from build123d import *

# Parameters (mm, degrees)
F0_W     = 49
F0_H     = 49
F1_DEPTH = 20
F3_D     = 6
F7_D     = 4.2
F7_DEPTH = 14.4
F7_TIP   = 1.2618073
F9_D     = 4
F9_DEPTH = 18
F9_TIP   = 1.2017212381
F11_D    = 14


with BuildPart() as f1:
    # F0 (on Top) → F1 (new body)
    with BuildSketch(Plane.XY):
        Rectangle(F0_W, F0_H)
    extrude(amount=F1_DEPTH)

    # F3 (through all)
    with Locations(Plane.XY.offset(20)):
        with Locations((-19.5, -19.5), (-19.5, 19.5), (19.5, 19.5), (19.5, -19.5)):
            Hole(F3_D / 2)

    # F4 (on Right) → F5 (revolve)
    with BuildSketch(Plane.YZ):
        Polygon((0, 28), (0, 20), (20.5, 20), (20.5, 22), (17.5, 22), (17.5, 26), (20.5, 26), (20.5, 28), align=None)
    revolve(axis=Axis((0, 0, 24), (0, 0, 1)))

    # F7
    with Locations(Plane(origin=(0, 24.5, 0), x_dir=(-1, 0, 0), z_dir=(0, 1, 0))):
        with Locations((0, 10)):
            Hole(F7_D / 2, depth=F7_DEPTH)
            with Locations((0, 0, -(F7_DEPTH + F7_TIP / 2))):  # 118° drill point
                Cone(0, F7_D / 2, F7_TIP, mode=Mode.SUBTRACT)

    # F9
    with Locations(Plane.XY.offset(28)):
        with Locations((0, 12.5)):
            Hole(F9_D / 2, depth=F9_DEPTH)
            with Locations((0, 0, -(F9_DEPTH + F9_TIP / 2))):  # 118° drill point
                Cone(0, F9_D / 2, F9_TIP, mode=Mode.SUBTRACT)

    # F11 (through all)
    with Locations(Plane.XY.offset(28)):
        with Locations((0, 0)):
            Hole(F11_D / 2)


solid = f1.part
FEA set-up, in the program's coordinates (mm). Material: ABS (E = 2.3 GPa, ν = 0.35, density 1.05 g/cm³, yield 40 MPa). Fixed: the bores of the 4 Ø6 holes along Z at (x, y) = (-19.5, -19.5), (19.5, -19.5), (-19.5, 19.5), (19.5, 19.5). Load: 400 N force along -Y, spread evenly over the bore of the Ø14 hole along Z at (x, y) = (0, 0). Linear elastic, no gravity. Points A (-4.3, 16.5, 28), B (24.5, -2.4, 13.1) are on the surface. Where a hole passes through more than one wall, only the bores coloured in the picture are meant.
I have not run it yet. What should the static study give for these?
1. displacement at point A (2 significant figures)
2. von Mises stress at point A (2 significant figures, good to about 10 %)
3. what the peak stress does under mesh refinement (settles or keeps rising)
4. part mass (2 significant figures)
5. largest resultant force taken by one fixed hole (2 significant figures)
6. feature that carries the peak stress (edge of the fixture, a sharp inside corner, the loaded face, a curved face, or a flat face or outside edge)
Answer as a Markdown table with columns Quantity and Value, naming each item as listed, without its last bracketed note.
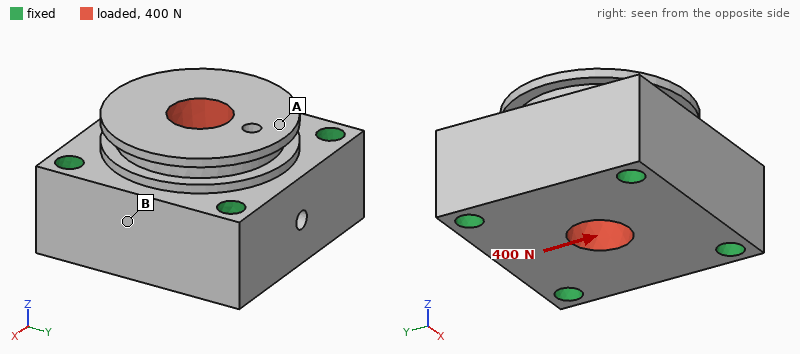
| Quantity | Value |
|---|---|
| displacement at point A | 5.3 µm |
| von Mises stress at point A | 0.29 MPa |
| what the peak stress does under mesh refinement | keeps rising |
| part mass | 53 g |
| largest resultant force taken by one fixed hole | 110 N |
| feature that carries the peak stress | edge of the fixture |
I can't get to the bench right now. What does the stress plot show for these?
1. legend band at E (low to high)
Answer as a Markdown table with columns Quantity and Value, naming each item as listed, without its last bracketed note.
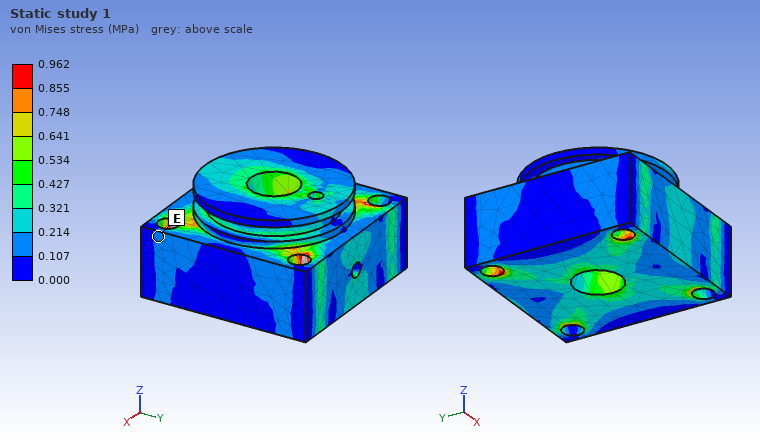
| Quantity | Value |
|---|---|
| legend band at E | 0.107 to 0.214 MPa |
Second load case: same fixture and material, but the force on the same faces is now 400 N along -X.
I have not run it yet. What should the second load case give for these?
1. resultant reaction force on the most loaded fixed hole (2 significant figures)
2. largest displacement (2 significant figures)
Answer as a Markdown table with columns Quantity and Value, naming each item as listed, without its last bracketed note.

| Quantity | Value |
|---|---|
| resultant reaction force on the most loaded fixed hole | 120 N |
| largest displacement | 6.6 µm |
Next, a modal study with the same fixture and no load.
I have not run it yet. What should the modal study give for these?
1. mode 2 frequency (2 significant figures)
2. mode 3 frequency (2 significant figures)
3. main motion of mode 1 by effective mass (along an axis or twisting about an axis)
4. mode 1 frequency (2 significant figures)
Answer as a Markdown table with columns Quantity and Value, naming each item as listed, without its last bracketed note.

| Quantity | Value |
|---|---|
| mode 2 frequency | 9000 Hz |
| mode 3 frequency | 9100 Hz |
| main motion of mode 1 by effective mass | along Z |
| mode 1 frequency | 7600 Hz |
